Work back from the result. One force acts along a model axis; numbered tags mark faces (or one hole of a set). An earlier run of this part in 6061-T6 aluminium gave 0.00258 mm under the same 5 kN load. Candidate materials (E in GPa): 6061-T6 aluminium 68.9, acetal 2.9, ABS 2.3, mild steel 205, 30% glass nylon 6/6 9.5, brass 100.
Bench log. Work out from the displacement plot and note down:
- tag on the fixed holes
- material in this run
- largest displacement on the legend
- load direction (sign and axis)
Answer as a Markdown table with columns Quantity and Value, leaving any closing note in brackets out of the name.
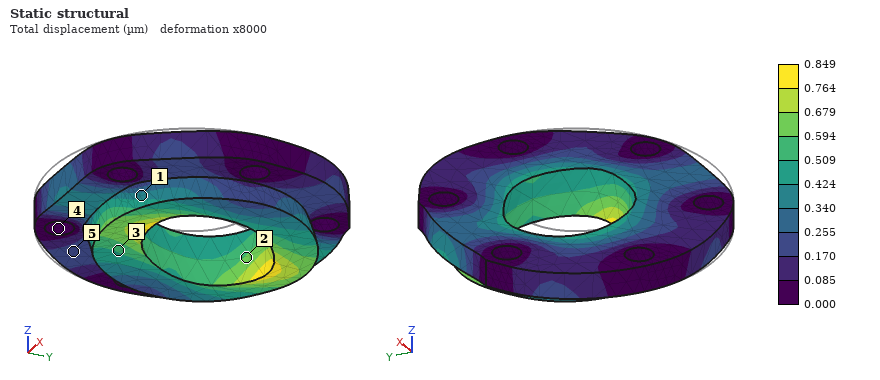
| Quantity | Value |
|---|---|
| tag on the fixed holes | 4 |
| material in this run | mild steel |
| largest displacement on the legend | 0.849 µm |
| load direction | +Y |
